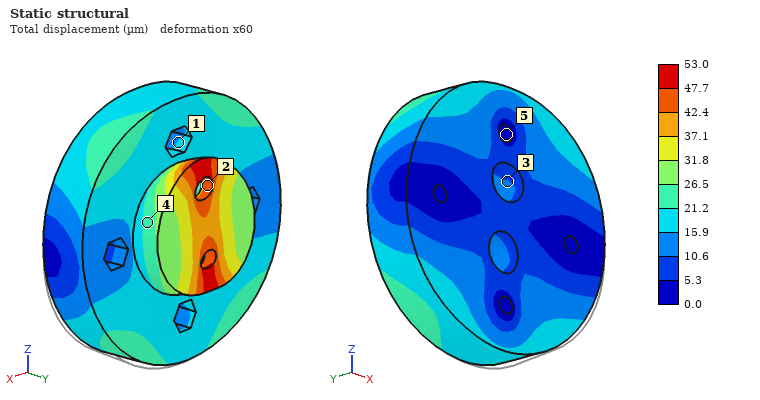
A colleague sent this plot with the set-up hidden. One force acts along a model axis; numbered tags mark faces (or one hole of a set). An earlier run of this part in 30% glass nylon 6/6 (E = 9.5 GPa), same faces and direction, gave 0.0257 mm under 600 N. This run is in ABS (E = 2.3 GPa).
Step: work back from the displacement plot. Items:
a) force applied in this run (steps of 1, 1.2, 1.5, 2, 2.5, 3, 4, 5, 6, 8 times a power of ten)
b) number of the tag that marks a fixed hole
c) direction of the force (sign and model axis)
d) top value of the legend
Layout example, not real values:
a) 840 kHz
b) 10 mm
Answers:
a) 300 N
b) 5
c) +Z
d) 53.0 µm
